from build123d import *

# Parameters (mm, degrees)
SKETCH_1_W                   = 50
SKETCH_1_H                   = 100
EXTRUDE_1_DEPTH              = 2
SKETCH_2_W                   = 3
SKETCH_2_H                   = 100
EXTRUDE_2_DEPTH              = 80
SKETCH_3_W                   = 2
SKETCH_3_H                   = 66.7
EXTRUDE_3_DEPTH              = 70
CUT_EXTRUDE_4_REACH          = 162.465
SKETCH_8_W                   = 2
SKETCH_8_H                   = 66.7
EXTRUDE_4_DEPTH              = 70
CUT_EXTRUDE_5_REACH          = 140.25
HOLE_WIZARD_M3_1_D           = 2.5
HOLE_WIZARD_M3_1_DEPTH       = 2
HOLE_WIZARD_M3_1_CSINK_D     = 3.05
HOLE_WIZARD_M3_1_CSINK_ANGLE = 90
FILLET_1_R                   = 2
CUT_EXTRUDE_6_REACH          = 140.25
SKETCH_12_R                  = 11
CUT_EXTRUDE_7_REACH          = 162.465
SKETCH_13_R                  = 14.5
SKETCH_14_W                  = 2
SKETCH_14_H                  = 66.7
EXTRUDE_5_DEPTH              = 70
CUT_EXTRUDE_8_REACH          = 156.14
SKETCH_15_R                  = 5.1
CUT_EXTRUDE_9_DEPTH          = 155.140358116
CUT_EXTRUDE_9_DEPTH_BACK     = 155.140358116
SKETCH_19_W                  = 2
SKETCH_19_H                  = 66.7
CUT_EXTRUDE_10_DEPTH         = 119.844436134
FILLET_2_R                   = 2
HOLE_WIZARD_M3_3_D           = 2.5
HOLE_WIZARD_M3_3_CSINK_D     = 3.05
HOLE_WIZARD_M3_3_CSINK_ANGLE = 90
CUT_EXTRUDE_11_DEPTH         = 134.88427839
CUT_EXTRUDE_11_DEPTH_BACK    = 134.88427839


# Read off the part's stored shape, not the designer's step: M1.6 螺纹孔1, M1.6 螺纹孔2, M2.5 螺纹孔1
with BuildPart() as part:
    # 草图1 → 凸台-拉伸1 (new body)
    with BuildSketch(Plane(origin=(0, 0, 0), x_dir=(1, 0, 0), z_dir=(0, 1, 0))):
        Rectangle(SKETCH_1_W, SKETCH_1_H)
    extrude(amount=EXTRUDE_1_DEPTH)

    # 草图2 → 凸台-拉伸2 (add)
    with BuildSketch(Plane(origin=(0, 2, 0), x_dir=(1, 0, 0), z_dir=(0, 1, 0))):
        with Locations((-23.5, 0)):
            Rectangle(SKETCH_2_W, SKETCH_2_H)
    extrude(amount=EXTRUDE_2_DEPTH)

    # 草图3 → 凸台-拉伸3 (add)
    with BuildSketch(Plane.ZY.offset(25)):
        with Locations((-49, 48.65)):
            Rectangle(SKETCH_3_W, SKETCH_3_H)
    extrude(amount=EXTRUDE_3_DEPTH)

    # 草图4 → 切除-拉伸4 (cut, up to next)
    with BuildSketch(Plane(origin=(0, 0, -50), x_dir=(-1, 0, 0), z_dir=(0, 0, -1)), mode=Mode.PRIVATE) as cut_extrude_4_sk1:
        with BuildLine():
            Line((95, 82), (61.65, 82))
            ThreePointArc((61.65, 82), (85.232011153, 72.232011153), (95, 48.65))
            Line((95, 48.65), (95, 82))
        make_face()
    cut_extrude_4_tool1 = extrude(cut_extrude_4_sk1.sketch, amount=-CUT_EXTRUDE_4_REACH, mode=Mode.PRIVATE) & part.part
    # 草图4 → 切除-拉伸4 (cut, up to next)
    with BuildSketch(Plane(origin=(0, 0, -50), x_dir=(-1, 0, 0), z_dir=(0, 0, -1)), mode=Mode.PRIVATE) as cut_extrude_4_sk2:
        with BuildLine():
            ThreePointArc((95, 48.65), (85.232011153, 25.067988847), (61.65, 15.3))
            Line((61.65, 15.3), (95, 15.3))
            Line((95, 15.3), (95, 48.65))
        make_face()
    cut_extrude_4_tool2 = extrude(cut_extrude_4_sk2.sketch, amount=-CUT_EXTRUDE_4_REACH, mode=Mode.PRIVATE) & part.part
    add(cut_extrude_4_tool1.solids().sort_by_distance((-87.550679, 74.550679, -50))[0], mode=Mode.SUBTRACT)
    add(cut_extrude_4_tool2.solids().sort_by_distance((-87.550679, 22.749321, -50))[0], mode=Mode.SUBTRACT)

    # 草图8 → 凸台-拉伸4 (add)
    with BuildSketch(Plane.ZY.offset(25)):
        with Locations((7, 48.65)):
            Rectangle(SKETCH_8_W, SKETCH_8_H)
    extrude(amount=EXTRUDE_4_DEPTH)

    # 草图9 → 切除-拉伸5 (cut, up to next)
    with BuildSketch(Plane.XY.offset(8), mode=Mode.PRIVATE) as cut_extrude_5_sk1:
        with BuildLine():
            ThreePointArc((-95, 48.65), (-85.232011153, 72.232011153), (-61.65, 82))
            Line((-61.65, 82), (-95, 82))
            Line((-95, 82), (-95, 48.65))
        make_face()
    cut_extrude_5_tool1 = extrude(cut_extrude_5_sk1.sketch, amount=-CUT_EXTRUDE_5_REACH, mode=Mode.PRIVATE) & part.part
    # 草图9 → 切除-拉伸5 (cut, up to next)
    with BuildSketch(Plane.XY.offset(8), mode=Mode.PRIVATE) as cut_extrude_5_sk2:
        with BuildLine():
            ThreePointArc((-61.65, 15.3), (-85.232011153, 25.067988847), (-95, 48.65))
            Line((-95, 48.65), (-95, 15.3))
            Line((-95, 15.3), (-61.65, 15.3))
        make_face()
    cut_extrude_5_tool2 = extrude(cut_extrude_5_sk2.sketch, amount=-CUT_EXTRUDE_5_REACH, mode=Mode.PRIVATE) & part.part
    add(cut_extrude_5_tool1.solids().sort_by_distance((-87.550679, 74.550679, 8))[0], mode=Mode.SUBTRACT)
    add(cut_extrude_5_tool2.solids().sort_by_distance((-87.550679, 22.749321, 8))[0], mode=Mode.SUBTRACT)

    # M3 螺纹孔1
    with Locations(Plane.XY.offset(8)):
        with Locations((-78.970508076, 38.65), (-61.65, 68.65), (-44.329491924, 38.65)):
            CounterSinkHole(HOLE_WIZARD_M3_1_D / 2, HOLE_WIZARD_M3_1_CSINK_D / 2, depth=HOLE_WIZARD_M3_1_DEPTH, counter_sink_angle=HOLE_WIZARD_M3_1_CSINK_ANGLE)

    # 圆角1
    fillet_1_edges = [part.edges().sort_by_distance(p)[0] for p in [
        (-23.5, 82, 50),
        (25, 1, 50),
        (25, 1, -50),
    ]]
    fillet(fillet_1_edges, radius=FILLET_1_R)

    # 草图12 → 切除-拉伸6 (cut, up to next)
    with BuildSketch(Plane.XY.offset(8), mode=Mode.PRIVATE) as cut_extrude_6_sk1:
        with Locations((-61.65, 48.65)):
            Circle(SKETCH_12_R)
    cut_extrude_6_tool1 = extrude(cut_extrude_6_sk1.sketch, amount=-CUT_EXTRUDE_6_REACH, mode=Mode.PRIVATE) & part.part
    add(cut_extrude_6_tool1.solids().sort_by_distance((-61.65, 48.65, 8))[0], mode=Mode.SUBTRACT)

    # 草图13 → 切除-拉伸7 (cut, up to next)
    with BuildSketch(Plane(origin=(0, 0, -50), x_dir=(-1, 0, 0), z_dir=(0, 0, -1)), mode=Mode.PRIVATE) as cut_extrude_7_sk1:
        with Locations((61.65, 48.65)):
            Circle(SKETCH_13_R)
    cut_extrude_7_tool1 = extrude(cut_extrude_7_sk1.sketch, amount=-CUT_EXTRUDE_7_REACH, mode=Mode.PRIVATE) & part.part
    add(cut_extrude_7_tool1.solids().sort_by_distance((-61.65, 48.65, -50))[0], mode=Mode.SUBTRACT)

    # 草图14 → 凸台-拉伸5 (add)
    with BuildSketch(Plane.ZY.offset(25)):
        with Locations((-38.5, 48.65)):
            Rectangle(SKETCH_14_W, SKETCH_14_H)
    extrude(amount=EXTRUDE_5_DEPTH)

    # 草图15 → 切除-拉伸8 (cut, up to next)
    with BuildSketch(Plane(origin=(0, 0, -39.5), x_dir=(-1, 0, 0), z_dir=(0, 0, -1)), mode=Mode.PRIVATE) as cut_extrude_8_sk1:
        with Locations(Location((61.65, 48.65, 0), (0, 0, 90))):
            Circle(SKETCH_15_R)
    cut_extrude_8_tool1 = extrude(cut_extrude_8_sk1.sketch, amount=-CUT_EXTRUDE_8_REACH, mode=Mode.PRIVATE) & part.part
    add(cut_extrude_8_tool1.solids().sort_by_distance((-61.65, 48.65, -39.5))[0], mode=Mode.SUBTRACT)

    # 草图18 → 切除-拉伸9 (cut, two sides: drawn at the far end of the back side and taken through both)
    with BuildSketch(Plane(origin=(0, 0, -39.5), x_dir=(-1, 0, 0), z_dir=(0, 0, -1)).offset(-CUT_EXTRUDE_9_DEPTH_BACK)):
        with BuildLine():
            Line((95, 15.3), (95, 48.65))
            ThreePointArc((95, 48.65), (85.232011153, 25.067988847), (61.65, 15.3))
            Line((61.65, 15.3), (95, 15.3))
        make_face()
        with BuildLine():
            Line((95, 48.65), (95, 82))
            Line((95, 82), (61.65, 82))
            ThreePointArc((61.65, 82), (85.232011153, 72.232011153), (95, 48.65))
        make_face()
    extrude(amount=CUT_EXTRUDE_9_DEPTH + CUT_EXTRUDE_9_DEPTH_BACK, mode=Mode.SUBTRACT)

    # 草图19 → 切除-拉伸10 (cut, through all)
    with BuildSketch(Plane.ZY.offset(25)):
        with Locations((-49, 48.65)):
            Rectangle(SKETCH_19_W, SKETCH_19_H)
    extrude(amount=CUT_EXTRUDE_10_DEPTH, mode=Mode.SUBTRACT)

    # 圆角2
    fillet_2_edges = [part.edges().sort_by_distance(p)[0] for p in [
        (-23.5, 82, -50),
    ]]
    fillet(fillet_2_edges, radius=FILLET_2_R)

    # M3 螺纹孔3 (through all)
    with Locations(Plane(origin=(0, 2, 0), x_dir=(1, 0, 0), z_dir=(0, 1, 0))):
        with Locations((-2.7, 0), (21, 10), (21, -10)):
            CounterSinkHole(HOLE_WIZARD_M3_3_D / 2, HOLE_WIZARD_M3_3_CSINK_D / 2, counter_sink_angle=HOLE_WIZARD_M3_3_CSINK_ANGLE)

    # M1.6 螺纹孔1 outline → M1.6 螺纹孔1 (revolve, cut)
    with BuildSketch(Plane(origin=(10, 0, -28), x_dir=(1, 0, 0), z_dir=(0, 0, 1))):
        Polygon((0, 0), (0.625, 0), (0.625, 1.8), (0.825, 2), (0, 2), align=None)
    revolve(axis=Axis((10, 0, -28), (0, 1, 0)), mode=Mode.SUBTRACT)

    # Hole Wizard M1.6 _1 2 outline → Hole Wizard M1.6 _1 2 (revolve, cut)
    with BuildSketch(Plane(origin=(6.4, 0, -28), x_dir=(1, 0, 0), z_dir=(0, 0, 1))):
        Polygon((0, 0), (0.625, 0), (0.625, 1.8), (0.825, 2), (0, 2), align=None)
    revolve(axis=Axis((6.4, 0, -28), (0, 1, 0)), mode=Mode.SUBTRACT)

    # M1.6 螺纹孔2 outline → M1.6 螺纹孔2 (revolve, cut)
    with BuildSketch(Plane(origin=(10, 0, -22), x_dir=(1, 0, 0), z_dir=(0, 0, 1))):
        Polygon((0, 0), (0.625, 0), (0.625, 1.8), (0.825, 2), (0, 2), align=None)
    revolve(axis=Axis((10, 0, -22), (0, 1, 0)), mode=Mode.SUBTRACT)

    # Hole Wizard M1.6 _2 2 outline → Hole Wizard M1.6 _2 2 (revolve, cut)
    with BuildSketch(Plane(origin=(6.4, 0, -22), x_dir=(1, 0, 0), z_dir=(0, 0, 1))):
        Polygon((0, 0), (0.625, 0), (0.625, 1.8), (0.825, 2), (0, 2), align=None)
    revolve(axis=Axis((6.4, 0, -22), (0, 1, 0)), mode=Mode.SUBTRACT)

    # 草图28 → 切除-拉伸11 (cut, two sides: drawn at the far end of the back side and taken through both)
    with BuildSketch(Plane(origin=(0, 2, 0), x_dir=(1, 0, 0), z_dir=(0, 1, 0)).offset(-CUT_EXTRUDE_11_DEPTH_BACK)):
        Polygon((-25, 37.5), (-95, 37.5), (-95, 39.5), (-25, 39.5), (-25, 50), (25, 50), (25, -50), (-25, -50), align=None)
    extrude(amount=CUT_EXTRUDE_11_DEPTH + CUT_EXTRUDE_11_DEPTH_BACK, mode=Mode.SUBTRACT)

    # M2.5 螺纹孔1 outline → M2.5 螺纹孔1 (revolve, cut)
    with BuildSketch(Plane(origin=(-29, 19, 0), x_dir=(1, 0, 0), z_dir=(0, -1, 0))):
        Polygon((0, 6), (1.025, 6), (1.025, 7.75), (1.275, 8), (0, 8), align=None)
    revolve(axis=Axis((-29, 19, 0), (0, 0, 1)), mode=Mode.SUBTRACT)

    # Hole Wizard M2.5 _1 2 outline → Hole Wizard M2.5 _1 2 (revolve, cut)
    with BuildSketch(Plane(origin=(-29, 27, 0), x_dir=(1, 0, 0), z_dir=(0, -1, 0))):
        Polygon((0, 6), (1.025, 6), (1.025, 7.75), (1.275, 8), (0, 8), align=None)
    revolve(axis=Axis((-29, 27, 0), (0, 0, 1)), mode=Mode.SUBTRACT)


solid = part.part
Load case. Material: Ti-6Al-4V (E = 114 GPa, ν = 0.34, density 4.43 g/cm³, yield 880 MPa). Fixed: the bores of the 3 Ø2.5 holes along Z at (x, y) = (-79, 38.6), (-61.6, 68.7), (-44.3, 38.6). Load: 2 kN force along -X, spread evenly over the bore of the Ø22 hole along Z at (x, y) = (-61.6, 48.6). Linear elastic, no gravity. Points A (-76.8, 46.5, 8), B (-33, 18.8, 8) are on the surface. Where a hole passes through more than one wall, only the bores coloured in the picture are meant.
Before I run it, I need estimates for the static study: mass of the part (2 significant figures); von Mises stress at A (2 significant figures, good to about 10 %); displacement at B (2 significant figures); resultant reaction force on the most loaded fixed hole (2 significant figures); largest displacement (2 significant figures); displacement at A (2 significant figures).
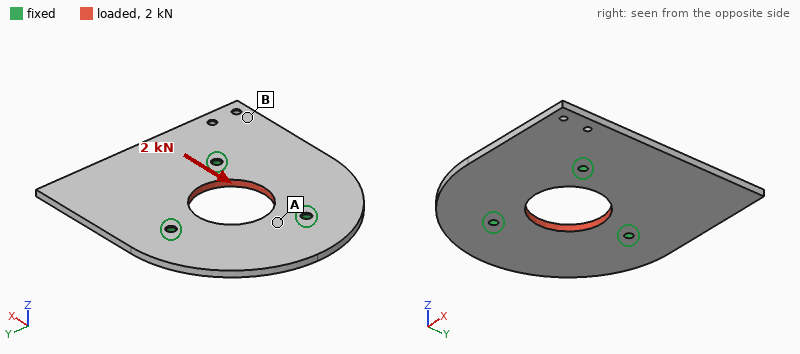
34 g
14 MPa
1.2 µm
720 N
4.2 µm
2.7 µm
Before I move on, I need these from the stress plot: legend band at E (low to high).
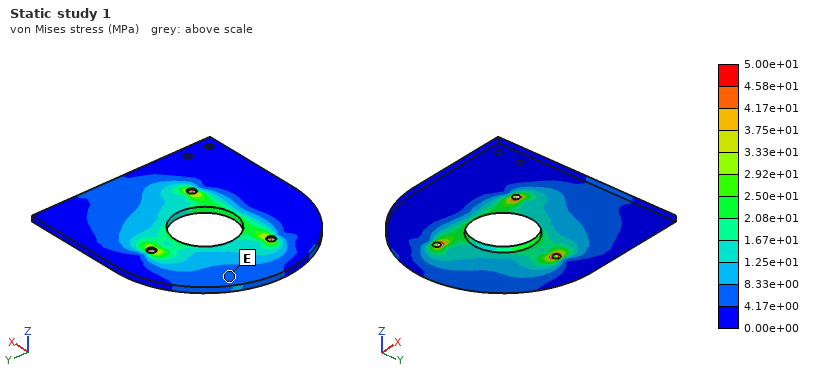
4.17e+00 to 8.33e+00 MPa
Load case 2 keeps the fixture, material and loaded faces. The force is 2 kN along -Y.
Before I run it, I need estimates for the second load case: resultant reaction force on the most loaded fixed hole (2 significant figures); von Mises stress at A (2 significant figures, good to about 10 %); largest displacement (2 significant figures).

700 N
18 MPa
4.6 µm
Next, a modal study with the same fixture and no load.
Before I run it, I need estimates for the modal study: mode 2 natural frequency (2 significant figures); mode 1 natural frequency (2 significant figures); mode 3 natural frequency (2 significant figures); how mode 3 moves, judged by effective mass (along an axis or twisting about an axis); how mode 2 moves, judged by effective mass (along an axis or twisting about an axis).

2500 Hz
1600 Hz
3000 Hz
along Z
along Z
